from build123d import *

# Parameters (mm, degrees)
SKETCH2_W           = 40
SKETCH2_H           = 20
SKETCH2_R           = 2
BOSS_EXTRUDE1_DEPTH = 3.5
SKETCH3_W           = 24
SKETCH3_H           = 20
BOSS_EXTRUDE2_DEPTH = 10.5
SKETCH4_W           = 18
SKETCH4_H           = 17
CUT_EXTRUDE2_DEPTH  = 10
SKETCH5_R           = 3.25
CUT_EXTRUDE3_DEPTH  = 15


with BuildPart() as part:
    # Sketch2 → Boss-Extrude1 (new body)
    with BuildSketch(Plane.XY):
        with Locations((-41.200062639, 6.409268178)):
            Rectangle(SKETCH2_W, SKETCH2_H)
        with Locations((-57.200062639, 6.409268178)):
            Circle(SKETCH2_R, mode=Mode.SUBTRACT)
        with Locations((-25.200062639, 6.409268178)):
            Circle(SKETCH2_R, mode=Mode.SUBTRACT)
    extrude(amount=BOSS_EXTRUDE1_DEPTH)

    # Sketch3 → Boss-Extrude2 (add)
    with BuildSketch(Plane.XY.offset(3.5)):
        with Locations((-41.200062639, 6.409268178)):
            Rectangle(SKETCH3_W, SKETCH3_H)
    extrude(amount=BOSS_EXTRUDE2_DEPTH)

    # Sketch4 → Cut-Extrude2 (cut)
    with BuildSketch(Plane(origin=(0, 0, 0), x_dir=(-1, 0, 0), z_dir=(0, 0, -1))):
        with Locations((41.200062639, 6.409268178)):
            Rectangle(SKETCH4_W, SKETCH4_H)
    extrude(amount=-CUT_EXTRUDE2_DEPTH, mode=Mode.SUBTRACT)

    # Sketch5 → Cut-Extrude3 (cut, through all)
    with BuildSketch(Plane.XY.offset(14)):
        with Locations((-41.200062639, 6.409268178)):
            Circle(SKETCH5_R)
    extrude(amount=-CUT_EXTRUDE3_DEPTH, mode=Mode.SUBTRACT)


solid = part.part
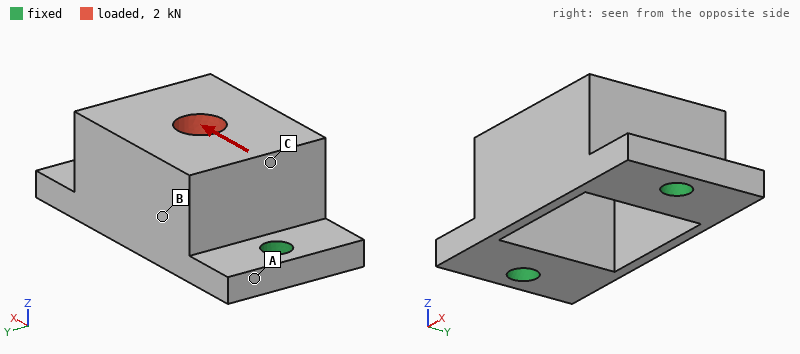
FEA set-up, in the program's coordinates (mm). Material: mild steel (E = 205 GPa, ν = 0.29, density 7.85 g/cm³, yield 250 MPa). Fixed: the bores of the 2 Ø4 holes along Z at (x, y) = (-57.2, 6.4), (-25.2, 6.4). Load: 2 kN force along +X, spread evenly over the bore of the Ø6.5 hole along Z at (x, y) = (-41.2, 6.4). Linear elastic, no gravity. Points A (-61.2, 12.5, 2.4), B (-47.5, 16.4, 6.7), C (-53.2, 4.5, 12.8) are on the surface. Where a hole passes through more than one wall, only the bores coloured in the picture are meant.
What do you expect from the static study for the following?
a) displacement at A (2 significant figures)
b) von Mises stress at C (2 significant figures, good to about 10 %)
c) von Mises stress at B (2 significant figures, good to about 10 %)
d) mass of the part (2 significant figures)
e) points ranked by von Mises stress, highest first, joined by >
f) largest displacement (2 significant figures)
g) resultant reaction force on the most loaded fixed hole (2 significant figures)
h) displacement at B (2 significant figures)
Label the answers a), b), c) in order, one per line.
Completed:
a) 1.2 µm
b) 20 MPa
c) 35 MPa
d) 36 g
e) B > C > A
f) 7.2 µm
g) 1.2 kN
h) 3.9 µm
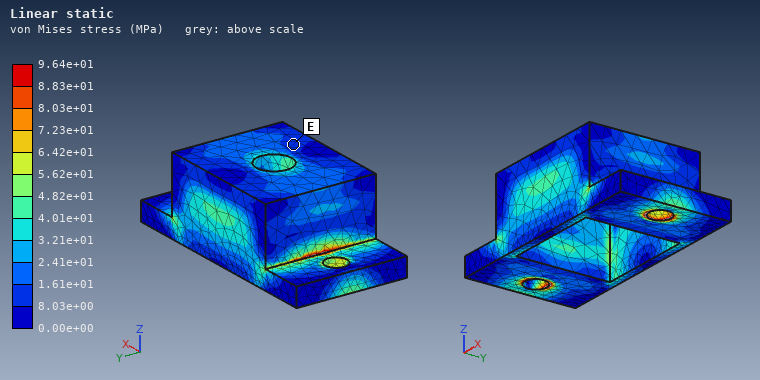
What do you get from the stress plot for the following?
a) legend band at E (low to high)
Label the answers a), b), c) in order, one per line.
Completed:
a) 8.03e+00 to 1.61e+01 MPa
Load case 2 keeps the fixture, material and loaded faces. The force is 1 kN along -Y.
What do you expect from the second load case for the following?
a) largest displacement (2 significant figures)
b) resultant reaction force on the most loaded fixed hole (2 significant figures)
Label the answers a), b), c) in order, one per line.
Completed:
a) 20 µm
b) 500 N
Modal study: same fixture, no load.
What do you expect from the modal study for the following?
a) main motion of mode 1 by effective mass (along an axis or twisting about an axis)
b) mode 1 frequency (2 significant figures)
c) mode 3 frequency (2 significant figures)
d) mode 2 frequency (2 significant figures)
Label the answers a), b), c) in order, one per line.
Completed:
a) along Y
b) 8500 Hz
c) 21 kHz
d) 21 kHz
